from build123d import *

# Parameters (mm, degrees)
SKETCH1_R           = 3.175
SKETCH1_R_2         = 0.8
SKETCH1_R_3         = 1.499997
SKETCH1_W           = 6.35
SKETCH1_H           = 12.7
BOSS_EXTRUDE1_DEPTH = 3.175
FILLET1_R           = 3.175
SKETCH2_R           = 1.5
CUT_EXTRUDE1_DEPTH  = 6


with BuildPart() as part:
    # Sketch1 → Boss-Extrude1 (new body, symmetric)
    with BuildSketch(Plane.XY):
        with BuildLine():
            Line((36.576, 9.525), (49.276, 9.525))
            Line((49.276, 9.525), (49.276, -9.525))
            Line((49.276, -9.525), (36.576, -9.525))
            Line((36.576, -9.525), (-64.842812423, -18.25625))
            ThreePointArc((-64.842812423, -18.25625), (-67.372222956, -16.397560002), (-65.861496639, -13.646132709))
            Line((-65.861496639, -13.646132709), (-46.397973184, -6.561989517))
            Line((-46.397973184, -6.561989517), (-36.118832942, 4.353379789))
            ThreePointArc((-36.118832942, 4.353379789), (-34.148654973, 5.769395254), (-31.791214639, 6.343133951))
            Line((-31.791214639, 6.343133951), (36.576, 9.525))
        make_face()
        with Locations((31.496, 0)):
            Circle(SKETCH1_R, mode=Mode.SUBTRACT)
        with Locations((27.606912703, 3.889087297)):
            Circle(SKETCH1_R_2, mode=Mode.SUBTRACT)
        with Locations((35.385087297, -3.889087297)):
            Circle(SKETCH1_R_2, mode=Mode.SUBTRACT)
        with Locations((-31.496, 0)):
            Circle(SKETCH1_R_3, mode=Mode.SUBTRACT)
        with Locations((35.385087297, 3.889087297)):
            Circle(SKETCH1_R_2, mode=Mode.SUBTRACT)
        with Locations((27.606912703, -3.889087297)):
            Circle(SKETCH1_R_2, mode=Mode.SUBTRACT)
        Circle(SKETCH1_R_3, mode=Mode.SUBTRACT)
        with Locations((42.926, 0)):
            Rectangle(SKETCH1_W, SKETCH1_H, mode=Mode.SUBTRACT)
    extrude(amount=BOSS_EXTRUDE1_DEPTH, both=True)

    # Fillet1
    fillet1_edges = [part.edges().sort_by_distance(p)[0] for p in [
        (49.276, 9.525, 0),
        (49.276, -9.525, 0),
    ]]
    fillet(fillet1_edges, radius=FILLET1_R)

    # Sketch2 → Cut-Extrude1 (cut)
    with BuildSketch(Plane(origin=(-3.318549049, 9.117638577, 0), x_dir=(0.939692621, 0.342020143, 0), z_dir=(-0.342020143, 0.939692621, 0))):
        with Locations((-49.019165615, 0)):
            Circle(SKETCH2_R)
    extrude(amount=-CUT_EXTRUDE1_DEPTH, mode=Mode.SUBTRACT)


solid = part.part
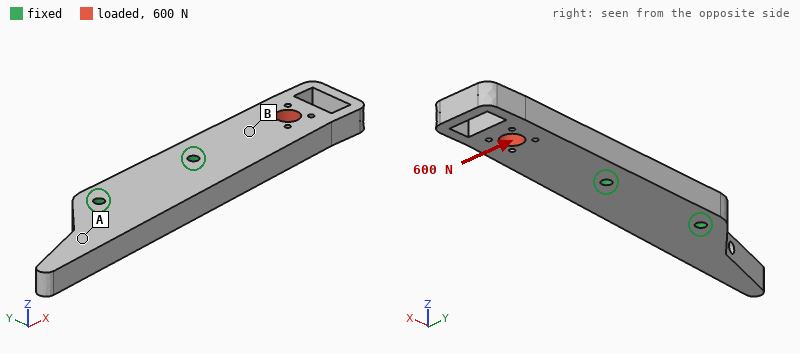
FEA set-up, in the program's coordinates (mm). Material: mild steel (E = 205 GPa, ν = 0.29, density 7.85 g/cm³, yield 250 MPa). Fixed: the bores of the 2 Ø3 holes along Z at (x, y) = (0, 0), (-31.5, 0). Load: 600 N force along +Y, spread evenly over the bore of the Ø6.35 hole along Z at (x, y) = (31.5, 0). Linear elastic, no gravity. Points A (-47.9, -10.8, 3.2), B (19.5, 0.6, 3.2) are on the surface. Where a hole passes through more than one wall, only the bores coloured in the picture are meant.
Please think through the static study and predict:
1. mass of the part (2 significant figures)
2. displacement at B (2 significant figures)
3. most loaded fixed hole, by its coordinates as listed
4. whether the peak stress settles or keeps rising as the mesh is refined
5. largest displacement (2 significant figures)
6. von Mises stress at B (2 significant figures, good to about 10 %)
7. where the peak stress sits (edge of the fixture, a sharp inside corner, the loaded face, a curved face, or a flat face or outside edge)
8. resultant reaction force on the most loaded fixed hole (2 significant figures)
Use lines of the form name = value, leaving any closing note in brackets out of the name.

mass of the part = 94 g
displacement at B = 8.8 µm
most loaded fixed hole, by its coordinates as listed = (0, 0)
whether the peak stress settles or keeps rising as the mesh is refined = keeps rising
largest displacement = 27 µm
von Mises stress at B = 13 MPa
where the peak stress sits = edge of the fixture
resultant reaction force on the most loaded fixed hole = 1.2 kN
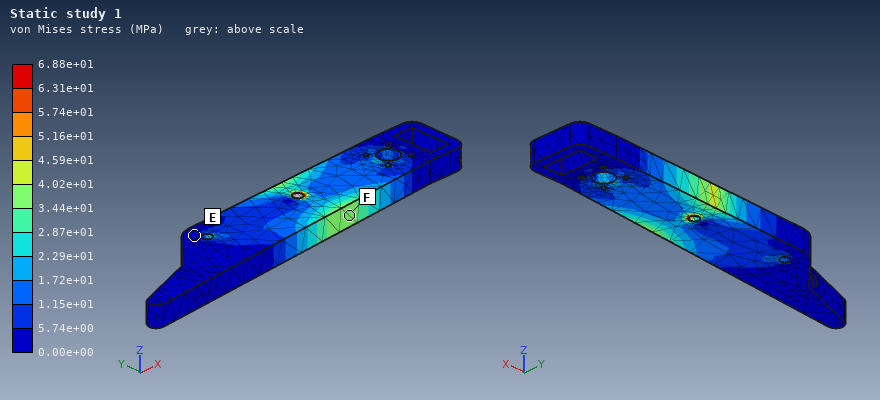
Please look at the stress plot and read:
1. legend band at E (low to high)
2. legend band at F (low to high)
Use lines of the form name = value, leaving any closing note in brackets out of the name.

legend band at E = 0.00e+00 to 5.74e+00 MPa
legend band at F = 3.44e+01 to 4.02e+01 MPa
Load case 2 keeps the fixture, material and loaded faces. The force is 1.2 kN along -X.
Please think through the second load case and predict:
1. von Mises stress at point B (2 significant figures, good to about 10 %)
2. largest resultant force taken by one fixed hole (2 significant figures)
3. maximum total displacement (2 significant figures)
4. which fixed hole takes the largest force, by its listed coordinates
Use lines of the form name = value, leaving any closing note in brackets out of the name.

von Mises stress at point B = 10 MPa
largest resultant force taken by one fixed hole = 1.1 kN
maximum total displacement = 3.4 µm
which fixed hole takes the largest force, by its listed coordinates = (0, 0)
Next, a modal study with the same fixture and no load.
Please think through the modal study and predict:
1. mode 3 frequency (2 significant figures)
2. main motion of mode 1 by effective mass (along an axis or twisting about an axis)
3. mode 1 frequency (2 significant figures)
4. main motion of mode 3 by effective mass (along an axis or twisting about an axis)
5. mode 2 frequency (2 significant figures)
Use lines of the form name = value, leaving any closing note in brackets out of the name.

mode 3 frequency = 5500 Hz
main motion of mode 1 by effective mass = along Z
mode 1 frequency = 2400 Hz
main motion of mode 3 by effective mass = along Y
mode 2 frequency = 4800 Hz
